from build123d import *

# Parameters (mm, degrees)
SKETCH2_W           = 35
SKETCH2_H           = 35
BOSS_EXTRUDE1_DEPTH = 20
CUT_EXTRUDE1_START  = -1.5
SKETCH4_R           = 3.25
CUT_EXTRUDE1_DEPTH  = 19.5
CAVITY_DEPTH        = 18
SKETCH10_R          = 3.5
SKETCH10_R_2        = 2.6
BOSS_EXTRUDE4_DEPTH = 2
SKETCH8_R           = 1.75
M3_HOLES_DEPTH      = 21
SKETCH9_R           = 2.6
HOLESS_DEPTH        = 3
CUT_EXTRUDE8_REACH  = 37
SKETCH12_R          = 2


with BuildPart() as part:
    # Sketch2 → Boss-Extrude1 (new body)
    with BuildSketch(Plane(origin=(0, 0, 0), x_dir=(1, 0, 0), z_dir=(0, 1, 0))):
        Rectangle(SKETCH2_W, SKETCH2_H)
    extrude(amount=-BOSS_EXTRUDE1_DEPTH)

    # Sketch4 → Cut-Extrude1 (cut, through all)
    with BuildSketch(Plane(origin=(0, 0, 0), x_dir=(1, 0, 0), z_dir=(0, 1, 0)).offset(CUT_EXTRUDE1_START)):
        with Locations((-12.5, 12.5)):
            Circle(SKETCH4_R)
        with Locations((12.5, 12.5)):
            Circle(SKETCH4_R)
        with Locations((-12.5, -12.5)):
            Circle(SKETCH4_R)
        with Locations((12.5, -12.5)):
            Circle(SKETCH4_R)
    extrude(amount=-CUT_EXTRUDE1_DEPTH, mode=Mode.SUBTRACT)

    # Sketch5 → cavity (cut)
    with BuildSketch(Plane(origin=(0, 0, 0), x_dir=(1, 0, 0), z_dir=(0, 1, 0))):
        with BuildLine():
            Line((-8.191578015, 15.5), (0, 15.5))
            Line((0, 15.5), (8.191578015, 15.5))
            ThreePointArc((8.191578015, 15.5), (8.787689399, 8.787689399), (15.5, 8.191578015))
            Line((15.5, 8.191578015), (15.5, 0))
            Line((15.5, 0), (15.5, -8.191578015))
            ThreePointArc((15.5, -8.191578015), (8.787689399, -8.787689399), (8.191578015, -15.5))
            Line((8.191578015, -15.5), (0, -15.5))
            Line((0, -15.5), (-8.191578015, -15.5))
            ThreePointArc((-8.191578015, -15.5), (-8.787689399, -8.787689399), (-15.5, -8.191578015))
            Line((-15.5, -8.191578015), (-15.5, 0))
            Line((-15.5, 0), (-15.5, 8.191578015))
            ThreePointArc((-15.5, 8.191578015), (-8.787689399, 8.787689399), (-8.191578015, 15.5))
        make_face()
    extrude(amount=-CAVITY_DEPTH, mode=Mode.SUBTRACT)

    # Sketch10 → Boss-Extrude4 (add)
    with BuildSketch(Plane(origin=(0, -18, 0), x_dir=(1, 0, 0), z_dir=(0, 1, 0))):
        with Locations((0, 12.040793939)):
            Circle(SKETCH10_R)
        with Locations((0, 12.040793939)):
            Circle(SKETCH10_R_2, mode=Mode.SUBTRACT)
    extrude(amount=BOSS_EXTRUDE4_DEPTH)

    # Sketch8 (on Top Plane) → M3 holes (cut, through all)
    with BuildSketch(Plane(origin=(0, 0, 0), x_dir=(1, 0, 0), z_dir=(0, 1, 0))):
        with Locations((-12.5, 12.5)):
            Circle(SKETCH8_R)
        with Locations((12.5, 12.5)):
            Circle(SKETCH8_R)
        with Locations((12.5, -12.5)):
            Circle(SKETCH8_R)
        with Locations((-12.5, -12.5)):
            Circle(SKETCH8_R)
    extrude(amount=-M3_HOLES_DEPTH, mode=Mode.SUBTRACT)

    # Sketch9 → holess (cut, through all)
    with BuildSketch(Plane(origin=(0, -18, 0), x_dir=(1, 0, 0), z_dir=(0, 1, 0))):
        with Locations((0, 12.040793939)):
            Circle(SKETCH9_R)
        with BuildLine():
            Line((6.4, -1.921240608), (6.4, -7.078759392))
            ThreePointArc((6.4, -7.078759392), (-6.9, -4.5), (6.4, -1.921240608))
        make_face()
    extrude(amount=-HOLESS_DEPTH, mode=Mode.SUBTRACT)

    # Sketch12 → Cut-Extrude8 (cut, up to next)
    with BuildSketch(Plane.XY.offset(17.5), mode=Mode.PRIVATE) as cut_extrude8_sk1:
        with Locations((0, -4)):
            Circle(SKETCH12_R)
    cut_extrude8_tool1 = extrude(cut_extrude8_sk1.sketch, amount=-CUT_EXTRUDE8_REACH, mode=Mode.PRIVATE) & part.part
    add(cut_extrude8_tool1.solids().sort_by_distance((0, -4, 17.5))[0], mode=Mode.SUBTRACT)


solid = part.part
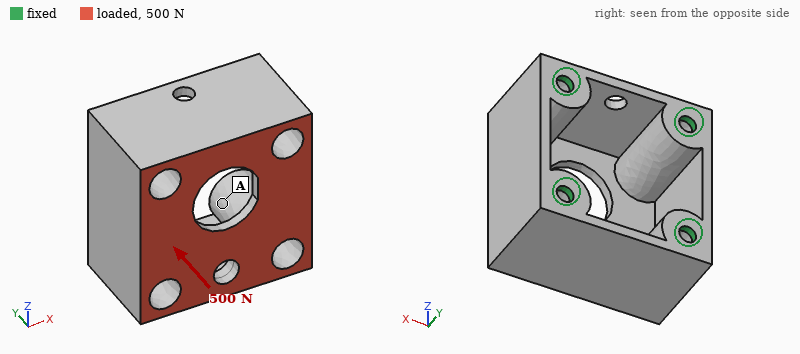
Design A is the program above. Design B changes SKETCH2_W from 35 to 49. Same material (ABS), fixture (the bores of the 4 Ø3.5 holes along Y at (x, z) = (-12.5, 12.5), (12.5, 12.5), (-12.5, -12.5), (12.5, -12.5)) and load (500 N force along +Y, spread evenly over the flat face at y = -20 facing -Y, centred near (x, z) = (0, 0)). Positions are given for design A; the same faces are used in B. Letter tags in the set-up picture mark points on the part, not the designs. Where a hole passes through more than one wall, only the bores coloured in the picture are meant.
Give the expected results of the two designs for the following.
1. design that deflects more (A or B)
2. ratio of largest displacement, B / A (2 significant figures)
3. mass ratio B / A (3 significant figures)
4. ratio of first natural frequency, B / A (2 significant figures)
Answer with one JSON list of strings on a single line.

["A", "0.64", "2.13", "0.62"]
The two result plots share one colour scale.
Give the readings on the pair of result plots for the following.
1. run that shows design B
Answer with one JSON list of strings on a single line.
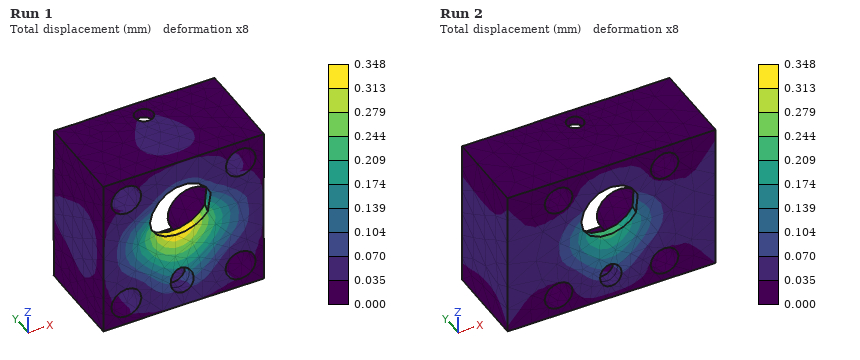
["Run 2"]
